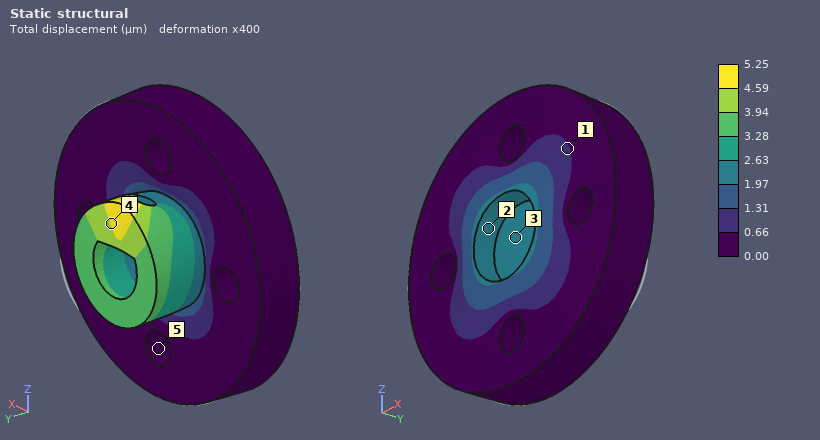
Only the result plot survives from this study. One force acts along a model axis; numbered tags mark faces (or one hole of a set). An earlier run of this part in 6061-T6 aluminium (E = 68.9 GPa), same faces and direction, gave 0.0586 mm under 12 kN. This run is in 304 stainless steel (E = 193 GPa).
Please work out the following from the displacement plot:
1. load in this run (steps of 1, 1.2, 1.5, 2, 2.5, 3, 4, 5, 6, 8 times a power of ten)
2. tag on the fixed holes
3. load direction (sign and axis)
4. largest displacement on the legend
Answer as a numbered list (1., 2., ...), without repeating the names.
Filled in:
1. 3 kN
2. 5
3. -Y
4. 5.25 µm
